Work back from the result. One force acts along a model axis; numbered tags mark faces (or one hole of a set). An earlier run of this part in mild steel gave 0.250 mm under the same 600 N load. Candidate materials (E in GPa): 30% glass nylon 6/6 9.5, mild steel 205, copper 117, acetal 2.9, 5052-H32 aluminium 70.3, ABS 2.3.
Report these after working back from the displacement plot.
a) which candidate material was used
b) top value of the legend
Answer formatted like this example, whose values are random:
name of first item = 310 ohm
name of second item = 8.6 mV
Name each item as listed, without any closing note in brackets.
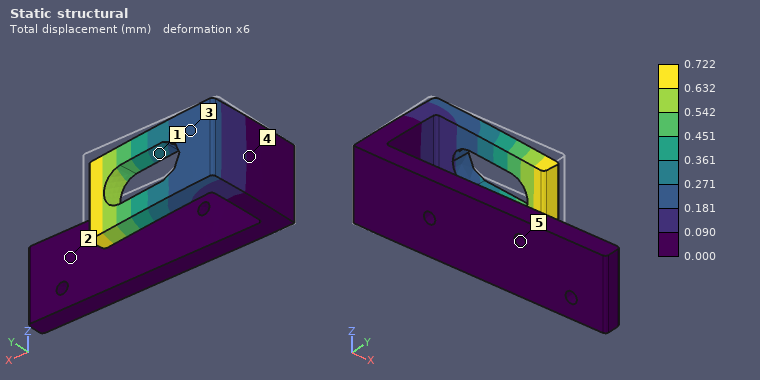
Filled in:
which candidate material was used = 5052-H32 aluminium
top value of the legend = 0.722 mm
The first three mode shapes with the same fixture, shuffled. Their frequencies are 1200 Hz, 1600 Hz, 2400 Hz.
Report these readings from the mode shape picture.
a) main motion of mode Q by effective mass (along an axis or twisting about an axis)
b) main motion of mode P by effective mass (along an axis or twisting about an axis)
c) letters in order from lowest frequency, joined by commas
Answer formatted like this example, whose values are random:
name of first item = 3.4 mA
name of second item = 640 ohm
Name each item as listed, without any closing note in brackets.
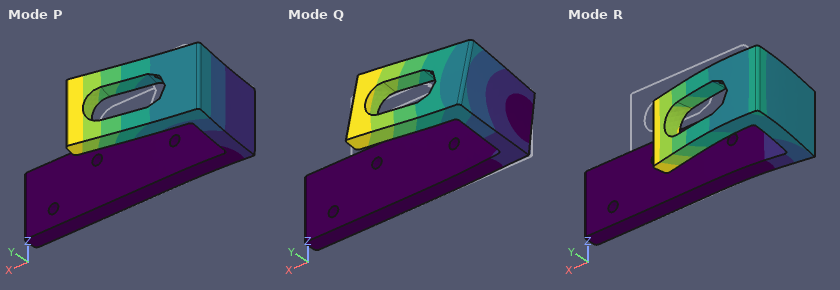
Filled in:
main motion of mode Q by effective mass = along Z
main motion of mode P by effective mass = along X
letters in order from lowest frequency, joined by commas = P, Q, R
